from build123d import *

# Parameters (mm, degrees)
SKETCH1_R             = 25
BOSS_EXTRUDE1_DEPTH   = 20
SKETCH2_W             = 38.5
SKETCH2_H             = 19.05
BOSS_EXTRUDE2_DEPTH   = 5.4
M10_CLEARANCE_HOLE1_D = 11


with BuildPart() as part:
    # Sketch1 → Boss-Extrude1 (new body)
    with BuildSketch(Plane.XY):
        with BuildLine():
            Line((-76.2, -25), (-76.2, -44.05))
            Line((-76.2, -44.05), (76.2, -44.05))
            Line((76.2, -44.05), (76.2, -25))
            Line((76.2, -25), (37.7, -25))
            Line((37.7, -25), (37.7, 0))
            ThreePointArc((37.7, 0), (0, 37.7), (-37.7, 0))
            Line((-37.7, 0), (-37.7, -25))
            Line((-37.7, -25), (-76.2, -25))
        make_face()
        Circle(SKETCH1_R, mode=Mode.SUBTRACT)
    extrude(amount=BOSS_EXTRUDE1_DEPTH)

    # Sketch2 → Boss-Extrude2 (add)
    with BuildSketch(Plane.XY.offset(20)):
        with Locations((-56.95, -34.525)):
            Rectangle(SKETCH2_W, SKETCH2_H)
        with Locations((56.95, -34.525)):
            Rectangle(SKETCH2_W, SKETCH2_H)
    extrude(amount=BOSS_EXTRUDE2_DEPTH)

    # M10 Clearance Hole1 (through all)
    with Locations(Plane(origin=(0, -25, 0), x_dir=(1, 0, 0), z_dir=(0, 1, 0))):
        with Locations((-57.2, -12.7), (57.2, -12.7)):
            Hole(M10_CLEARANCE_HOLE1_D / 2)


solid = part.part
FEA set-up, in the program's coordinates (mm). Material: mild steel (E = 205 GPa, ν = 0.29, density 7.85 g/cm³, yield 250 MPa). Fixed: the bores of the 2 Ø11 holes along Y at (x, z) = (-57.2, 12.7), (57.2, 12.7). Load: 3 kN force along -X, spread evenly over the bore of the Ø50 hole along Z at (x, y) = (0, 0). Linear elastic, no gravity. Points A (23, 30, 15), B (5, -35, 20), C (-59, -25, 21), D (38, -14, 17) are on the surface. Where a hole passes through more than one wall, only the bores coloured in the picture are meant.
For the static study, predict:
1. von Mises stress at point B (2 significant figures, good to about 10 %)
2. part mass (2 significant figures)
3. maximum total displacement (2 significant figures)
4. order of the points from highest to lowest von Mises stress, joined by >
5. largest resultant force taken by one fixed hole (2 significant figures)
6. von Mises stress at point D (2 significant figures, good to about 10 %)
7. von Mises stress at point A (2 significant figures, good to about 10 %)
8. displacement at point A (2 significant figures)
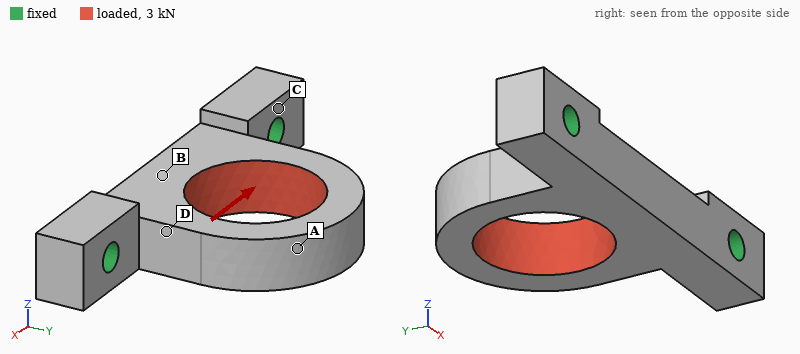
5.4 MPa
830 g
11 µm
D > A > B > C
1.9 kN
16 MPa
9.6 MPa
11 µm
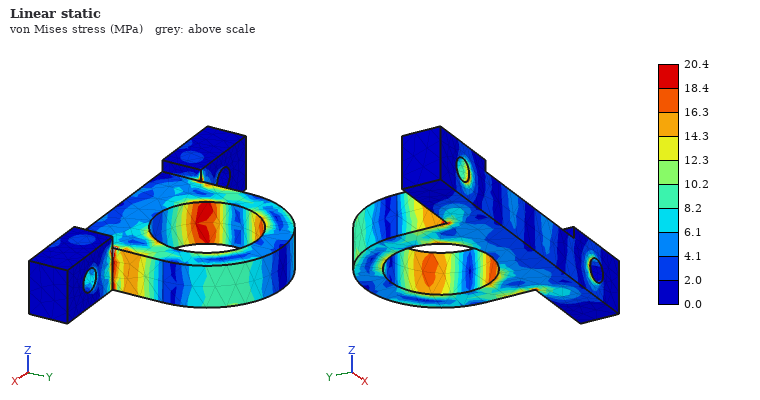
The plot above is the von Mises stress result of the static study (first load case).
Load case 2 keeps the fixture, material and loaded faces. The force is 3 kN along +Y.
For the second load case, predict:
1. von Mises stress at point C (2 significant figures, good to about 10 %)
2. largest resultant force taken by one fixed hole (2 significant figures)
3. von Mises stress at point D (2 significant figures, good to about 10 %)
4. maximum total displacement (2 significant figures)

3.4 MPa
1.5 kN
8.8 MPa
4.1 µm
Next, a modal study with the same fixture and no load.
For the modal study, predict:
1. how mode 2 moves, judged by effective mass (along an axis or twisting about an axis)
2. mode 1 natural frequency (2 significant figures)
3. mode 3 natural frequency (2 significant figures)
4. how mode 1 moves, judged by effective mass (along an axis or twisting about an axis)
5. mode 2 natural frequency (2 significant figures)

along X
2000 Hz
5500 Hz
along Z
4500 Hz
